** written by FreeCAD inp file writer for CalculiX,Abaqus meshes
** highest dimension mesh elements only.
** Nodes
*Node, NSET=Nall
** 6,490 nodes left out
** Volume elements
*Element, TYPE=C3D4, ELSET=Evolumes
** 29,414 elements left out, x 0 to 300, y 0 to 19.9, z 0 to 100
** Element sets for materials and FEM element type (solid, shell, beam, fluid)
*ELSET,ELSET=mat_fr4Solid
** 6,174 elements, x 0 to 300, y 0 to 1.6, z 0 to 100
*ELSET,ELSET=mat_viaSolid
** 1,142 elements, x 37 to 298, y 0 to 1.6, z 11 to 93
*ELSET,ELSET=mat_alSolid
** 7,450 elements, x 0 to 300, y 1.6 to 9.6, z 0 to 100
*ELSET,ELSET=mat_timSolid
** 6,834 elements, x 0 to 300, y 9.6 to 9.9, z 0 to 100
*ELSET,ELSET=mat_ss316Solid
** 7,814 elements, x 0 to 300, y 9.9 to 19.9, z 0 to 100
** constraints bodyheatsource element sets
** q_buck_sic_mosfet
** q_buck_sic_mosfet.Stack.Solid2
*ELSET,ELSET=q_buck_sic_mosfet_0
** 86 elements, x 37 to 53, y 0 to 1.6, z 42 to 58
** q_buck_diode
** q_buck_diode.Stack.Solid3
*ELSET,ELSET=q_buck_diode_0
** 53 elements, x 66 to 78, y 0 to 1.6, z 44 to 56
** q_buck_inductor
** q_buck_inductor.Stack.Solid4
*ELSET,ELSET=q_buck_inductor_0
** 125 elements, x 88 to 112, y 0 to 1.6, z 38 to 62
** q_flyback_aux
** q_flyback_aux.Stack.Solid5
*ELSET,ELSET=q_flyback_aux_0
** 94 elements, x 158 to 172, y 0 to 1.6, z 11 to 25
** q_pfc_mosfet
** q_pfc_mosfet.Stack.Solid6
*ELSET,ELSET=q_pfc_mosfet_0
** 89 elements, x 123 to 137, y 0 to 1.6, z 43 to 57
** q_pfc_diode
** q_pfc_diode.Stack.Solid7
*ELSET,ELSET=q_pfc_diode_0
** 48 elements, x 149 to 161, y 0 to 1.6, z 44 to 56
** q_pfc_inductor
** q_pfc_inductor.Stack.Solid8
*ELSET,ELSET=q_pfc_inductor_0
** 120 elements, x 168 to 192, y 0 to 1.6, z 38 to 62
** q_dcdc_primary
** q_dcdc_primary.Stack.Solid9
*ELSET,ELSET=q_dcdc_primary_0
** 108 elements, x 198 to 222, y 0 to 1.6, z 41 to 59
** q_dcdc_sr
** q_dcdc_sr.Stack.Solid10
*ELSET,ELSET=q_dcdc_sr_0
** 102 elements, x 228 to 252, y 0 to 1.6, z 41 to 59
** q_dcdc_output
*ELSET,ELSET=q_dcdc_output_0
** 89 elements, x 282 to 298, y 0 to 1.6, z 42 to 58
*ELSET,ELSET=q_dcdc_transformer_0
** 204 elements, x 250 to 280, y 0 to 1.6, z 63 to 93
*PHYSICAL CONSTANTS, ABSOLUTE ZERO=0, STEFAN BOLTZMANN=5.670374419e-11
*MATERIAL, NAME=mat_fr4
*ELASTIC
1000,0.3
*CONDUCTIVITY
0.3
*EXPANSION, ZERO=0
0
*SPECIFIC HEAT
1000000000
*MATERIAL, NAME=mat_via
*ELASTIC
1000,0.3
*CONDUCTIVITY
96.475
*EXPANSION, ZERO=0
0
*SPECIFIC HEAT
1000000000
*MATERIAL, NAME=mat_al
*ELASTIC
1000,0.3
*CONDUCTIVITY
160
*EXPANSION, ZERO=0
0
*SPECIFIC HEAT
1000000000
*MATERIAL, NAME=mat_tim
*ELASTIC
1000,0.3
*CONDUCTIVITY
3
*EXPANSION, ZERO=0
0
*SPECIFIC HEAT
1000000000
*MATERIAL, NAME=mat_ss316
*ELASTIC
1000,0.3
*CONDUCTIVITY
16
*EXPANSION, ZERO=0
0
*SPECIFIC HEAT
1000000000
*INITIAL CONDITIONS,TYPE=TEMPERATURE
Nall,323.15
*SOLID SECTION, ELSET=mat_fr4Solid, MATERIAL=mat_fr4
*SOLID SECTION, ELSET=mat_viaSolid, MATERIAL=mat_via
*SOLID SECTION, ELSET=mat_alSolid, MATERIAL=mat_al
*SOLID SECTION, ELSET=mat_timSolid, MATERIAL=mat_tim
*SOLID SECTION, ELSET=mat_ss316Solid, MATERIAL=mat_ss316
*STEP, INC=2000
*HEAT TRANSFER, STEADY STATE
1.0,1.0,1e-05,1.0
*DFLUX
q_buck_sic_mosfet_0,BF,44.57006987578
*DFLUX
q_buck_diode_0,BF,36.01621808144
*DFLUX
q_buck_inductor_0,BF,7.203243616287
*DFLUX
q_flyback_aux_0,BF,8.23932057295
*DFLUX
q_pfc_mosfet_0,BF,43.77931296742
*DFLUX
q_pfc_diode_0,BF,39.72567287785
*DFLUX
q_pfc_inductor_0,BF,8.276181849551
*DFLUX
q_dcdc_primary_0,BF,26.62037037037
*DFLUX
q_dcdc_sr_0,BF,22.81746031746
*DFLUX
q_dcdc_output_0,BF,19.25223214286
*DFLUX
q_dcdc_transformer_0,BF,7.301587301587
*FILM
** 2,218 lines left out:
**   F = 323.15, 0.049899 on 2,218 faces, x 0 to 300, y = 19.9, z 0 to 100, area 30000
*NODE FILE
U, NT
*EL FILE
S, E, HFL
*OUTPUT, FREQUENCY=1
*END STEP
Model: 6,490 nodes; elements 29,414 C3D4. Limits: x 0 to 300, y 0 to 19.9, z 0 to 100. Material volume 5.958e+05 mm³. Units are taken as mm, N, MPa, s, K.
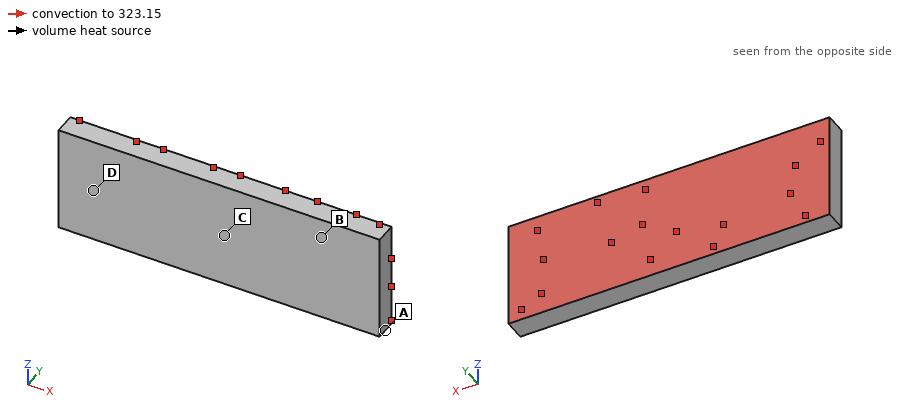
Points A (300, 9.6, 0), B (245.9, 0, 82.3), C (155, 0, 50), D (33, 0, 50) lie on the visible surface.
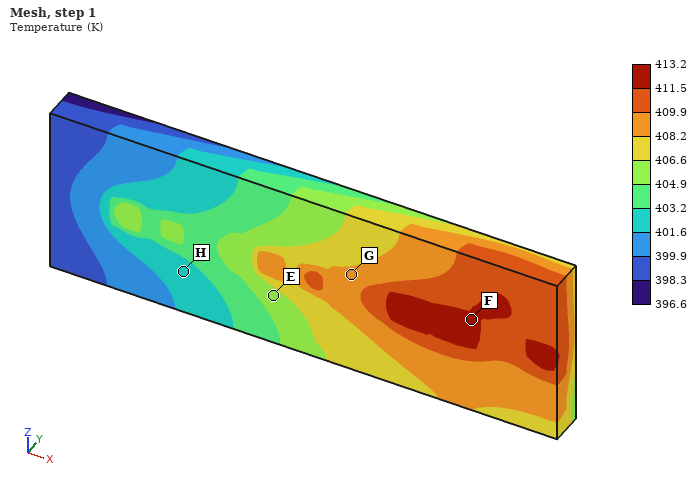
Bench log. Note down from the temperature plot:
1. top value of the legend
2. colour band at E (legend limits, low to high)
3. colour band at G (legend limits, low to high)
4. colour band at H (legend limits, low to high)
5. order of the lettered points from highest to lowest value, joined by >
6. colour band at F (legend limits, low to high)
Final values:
413.2 K
404.9 to 406.6 K
408.2 to 409.9 K
401.6 to 403.2 K
F > G > E > H
411.5 to 413.2 K
